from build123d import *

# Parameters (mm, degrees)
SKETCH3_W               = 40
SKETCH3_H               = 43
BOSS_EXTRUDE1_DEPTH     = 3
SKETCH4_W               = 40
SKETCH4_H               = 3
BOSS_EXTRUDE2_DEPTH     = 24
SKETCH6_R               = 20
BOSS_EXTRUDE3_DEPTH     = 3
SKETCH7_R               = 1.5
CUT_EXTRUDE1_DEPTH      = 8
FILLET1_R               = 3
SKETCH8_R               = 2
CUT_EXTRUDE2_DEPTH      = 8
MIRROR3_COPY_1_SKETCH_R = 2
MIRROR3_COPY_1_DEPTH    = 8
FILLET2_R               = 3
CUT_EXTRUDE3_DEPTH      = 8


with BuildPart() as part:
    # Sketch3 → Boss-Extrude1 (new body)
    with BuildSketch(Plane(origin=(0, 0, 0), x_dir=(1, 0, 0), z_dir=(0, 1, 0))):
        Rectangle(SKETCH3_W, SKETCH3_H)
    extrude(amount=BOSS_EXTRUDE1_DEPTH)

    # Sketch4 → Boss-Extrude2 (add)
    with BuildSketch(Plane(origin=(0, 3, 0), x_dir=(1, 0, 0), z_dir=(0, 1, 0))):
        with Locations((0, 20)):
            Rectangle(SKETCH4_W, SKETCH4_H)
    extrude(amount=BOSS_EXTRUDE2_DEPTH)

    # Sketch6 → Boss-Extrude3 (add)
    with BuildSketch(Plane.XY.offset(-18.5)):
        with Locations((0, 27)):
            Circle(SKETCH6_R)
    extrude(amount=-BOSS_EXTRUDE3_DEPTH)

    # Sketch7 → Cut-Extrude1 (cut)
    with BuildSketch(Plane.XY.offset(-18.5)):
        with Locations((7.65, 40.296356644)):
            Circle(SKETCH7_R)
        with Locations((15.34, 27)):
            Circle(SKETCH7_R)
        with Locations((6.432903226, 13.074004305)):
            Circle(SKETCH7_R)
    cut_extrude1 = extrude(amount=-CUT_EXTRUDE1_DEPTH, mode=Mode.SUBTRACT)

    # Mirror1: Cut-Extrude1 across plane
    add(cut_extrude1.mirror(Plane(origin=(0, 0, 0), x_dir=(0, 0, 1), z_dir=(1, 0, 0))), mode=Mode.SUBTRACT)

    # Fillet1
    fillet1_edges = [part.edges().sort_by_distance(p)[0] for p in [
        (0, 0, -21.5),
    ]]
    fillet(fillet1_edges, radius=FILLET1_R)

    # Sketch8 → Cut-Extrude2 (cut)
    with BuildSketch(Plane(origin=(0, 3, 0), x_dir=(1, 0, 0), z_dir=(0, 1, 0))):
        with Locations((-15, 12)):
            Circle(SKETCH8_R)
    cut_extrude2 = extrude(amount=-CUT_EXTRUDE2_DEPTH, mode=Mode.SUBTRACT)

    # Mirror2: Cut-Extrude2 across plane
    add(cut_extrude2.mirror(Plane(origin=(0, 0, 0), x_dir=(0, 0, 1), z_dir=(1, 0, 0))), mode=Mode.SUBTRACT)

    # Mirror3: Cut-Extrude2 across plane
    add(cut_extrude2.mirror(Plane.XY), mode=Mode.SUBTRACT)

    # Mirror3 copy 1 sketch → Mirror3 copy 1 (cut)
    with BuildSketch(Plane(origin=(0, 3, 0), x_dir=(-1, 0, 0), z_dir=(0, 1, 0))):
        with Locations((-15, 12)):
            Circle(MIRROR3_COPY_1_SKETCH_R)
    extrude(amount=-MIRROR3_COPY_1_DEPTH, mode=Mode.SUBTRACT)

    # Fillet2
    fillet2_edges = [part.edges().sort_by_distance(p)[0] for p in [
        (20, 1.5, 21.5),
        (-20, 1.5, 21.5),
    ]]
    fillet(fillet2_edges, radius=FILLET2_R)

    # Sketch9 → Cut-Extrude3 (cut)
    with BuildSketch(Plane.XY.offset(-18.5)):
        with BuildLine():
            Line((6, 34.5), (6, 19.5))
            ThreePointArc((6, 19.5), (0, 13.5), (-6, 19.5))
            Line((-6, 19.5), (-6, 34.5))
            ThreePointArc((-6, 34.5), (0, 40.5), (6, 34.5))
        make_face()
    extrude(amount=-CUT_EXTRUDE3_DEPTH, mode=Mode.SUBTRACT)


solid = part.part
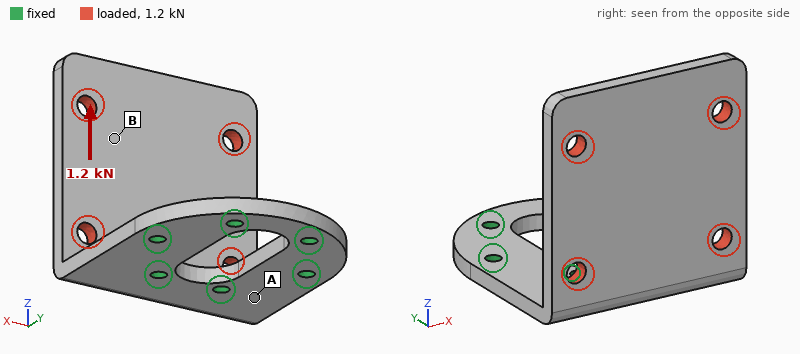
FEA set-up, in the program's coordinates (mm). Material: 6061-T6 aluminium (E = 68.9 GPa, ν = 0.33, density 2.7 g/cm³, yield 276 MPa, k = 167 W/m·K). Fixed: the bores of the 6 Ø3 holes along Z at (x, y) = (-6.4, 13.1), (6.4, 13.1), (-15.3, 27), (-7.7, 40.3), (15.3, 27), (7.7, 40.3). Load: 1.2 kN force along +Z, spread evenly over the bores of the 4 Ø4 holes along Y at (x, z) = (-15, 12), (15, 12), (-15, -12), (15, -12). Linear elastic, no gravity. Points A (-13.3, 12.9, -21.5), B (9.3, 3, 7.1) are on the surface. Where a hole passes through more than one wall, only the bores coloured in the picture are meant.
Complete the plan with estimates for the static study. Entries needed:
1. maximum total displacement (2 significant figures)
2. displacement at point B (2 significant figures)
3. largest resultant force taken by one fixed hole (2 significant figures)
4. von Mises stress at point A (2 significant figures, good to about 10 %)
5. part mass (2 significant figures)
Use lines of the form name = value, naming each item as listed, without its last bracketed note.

maximum total displacement = 0.59 mm
displacement at point B = 0.39 mm
largest resultant force taken by one fixed hole = 730 N
von Mises stress at point A = 100 MPa
part mass = 23 g
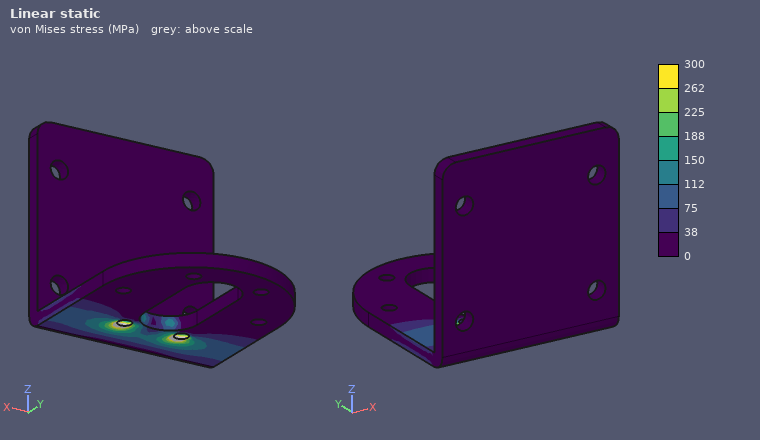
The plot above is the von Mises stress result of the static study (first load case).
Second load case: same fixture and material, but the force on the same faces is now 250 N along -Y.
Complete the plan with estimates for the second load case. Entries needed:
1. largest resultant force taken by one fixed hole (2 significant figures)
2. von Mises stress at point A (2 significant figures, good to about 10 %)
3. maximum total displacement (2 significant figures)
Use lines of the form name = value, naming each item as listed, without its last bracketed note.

largest resultant force taken by one fixed hole = 120 N
von Mises stress at point A = 45 MPa
maximum total displacement = 0.70 mm
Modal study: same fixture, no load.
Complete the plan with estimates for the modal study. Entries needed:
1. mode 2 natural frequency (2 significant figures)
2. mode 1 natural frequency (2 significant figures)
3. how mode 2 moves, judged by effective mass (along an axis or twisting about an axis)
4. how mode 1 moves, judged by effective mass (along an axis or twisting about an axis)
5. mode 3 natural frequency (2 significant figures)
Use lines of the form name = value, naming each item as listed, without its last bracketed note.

mode 2 natural frequency = 2100 Hz
mode 1 natural frequency = 1000 Hz
how mode 2 moves, judged by effective mass = along X
how mode 1 moves, judged by effective mass = along Y
mode 3 natural frequency = 3400 Hz
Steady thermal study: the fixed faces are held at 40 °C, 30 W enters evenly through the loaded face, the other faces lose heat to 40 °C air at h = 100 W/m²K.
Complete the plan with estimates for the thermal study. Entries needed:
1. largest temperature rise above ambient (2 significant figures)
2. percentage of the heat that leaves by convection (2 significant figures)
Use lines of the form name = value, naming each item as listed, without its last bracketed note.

largest temperature rise above ambient = 37 K
percentage of the heat that leaves by convection = 35 %
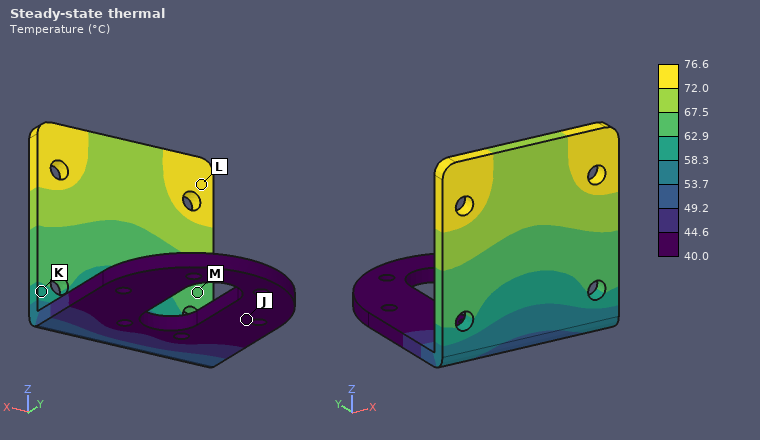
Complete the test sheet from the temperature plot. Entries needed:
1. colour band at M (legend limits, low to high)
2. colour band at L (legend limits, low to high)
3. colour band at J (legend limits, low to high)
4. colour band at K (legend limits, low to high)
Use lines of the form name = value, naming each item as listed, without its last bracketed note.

colour band at M = 62.9 to 67.5 °C
colour band at L = 72.0 to 76.6 °C
colour band at J = 40.0 to 44.6 °C
colour band at K = 58.3 to 62.9 °C
